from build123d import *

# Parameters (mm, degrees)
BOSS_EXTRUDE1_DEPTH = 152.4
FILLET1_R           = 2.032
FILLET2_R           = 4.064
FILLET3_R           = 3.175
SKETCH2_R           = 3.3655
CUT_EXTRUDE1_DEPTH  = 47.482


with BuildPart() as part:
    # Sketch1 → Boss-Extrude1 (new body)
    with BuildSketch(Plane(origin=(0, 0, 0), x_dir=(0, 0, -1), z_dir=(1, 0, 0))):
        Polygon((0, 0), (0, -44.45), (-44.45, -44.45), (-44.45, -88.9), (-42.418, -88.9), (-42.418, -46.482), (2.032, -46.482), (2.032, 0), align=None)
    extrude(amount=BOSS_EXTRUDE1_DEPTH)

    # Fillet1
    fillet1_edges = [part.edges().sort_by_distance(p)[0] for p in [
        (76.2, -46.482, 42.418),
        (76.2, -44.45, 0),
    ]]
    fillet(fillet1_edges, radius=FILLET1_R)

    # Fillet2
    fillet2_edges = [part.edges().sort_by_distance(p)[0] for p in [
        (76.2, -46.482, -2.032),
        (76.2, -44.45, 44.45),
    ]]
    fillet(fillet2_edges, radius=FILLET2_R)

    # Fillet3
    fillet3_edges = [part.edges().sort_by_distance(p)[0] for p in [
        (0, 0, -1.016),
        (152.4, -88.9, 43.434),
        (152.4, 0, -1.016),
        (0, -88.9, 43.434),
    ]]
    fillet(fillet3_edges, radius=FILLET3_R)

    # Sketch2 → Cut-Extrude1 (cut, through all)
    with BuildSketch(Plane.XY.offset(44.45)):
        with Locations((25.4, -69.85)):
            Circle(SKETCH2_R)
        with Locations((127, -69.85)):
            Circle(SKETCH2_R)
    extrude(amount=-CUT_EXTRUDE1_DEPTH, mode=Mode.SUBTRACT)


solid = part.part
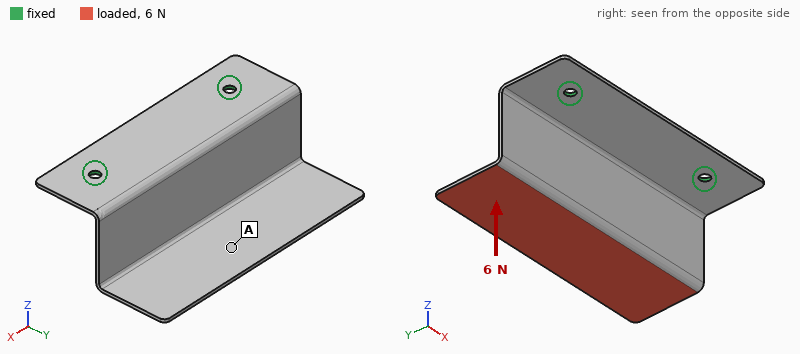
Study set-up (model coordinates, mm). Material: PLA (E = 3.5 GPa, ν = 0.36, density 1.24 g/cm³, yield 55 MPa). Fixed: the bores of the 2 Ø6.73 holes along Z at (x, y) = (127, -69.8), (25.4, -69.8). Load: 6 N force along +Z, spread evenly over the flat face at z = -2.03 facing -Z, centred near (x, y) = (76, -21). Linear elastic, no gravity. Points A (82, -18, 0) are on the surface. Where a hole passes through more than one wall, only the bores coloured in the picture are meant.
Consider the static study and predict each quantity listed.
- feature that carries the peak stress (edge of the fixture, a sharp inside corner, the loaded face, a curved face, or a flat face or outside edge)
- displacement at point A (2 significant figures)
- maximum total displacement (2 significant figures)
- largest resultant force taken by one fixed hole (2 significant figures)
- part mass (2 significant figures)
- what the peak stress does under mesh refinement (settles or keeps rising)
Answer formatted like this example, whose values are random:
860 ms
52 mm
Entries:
edge of the fixture
1.6 mm
2.1 mm
3.0 N
50 g
keeps rising
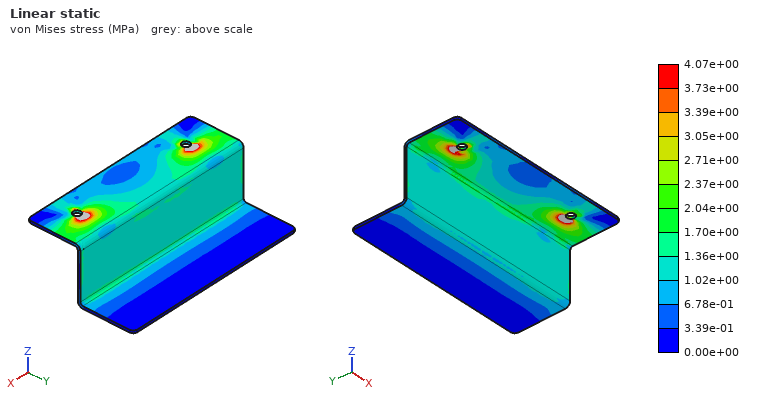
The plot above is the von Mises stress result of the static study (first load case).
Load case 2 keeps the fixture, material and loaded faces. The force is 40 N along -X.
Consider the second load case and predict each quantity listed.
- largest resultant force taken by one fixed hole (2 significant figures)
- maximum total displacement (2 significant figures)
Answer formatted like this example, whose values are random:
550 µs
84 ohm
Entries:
32 N
1.8 mm
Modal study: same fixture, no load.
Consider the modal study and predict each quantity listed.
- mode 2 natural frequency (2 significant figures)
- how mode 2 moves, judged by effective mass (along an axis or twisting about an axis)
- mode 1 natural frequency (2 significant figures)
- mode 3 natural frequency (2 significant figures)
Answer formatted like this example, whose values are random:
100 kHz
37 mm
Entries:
110 Hz
twisting about Z
57 Hz
240 Hz
